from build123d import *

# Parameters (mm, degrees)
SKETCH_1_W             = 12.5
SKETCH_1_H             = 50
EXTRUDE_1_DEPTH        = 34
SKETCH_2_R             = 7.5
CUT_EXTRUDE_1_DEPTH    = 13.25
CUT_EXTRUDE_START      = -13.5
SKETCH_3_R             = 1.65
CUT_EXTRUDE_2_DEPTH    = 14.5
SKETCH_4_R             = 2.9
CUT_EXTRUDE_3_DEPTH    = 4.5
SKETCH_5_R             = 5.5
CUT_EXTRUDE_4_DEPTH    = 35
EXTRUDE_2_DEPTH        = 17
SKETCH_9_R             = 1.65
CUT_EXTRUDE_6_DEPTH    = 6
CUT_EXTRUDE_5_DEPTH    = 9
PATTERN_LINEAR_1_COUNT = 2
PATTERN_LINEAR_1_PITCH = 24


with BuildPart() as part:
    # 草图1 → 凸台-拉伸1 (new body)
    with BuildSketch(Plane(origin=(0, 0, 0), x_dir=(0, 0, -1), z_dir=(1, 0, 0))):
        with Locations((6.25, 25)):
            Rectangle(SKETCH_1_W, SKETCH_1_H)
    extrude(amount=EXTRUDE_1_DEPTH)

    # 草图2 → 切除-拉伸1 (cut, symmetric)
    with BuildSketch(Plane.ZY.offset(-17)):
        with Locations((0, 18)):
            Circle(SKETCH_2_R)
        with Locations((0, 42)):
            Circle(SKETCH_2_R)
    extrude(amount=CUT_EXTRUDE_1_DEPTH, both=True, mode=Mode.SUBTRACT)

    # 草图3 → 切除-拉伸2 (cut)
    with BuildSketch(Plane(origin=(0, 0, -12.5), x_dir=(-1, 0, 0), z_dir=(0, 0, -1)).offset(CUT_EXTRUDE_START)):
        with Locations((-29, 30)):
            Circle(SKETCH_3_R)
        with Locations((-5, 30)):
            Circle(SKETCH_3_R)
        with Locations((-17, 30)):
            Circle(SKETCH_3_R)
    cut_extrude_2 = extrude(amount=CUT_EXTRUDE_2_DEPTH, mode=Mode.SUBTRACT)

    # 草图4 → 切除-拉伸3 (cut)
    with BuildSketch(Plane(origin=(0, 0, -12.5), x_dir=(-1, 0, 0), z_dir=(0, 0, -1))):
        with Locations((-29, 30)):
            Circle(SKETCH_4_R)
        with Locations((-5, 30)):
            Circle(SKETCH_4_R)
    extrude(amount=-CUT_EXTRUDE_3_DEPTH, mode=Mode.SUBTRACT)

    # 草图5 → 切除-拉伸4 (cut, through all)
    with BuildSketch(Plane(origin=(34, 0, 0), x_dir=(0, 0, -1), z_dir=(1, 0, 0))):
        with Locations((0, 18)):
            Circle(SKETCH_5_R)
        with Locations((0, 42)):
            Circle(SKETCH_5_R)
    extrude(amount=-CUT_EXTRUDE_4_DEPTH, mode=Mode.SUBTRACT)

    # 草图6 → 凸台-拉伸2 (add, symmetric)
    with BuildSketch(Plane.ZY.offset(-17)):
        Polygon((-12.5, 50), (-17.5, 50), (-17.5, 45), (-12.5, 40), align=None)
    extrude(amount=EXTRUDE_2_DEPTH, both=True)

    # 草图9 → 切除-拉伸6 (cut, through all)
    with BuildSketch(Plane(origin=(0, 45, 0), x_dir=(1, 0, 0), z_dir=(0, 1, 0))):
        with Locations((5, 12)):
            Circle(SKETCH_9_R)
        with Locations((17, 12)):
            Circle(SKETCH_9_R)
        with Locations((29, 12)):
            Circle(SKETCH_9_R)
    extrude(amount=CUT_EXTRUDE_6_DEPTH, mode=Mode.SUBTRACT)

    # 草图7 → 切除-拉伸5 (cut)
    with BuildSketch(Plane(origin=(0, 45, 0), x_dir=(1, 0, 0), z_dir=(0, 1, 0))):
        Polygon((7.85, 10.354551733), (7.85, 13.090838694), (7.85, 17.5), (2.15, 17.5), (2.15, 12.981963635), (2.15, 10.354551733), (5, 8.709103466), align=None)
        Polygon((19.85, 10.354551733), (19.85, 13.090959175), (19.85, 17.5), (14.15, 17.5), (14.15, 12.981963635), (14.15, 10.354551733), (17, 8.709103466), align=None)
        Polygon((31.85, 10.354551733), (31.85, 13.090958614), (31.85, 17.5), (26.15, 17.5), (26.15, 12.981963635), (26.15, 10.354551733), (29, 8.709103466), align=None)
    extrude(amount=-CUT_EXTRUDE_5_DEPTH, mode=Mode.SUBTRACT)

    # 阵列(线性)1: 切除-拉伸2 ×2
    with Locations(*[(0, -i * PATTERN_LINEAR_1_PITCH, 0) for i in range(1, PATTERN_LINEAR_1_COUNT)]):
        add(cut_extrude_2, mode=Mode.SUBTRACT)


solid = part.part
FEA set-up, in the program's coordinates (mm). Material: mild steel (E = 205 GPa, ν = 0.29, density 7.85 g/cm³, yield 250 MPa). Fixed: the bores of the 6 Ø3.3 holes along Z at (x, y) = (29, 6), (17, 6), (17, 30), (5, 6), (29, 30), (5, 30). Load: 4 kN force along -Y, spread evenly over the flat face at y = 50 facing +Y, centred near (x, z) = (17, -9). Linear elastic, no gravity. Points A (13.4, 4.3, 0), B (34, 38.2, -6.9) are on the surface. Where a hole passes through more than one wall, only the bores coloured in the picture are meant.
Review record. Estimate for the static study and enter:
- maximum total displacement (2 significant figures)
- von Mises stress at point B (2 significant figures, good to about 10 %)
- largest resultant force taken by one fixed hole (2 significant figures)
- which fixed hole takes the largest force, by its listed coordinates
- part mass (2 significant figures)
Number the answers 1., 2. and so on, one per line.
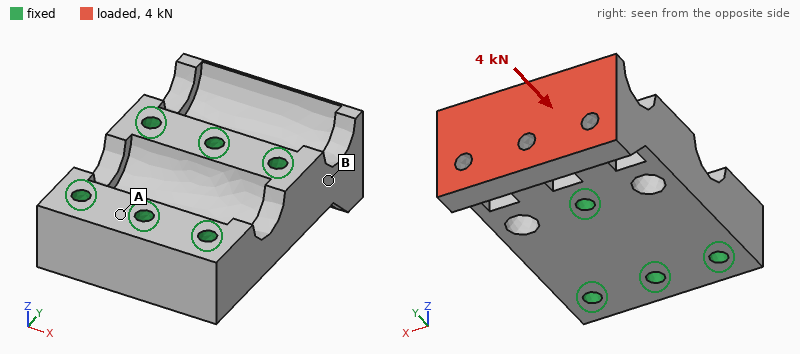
1. 23 µm
2. 25 MPa
3. 1.5 kN
4. (17, 30)
5. 120 g
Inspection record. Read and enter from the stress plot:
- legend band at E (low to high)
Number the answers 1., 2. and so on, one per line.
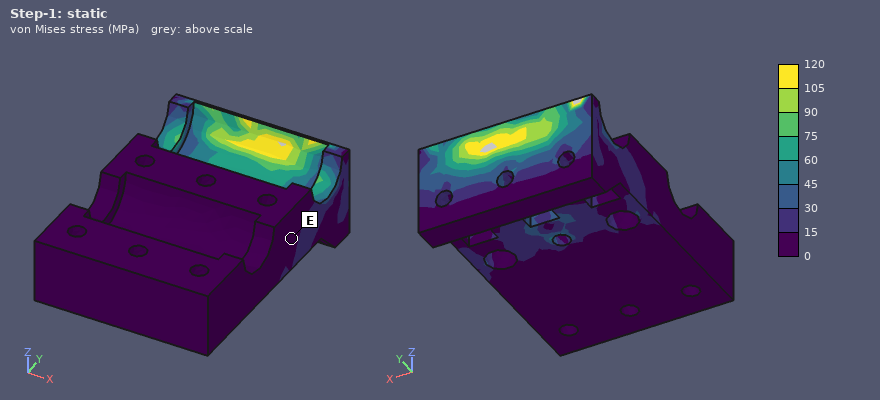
1. 0 to 15 MPa
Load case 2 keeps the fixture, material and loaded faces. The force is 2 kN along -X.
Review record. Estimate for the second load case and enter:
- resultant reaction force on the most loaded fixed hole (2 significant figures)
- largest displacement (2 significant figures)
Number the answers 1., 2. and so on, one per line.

1. 1.3 kN
2. 9.1 µm
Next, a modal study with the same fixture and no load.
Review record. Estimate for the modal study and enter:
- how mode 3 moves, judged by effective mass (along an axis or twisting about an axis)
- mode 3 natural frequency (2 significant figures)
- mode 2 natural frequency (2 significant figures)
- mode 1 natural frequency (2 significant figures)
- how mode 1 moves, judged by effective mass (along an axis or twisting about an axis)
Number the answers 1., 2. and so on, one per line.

1. along X
2. 22 kHz
3. 16 kHz
4. 11 kHz
5. along Z
